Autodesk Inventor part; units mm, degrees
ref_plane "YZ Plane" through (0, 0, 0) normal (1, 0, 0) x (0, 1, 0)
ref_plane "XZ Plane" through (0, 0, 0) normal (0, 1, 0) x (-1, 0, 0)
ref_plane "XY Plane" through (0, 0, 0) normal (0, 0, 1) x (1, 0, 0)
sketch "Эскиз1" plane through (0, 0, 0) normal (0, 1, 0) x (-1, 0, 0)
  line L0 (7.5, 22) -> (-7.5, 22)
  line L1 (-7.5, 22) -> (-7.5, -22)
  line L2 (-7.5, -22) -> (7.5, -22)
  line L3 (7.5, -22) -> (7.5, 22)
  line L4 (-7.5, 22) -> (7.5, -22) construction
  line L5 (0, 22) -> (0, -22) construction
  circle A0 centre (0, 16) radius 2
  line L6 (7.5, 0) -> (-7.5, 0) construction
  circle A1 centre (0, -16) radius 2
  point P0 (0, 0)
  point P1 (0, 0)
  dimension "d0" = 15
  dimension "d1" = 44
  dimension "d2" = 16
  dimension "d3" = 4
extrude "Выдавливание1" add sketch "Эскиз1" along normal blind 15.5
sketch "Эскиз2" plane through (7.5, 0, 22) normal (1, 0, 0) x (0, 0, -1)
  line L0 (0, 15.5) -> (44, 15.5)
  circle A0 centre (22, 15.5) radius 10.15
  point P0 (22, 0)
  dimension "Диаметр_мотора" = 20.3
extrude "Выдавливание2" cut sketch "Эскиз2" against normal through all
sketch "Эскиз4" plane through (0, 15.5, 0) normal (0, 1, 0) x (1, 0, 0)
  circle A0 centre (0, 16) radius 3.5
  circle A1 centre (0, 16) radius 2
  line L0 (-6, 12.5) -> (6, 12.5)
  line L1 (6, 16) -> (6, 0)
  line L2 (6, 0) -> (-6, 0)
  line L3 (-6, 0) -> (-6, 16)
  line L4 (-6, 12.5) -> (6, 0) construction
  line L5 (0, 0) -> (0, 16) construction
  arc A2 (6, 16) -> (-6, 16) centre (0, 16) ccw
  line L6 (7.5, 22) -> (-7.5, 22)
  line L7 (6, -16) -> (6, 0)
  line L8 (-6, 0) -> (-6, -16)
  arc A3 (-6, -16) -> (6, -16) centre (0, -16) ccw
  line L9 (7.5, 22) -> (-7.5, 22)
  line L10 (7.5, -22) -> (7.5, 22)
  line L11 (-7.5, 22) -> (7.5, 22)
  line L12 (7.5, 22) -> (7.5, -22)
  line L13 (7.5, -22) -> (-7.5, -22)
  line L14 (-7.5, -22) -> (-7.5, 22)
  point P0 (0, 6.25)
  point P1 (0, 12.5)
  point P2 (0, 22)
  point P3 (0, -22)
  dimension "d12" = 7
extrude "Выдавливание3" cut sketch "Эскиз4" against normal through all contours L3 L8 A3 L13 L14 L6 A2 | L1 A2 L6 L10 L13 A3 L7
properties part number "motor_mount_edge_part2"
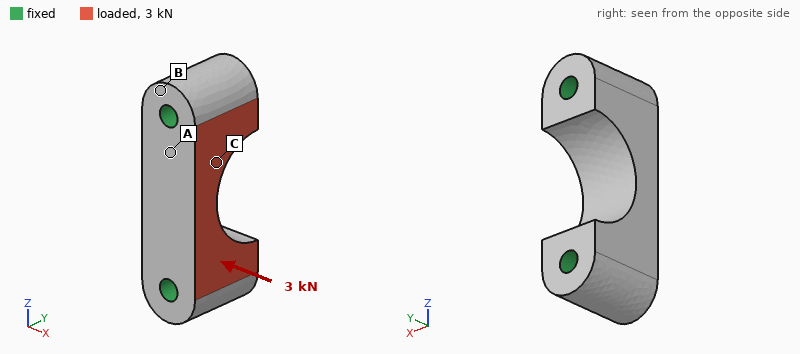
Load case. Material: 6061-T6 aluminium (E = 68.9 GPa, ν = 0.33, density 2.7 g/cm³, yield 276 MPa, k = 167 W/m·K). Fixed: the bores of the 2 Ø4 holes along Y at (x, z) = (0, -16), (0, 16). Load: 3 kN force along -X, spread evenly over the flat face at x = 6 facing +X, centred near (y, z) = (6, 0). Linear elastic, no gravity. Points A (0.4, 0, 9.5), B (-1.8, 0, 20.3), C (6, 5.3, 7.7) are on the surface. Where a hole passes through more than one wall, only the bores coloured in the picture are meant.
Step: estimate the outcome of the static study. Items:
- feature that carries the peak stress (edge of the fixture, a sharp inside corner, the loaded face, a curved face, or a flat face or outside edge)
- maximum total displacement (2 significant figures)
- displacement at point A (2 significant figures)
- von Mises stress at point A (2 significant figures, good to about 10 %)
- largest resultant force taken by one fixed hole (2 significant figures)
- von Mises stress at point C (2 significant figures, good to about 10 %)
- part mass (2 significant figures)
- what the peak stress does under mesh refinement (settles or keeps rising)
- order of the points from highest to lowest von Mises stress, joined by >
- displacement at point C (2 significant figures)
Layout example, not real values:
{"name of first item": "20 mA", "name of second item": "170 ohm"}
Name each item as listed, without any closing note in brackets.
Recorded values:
{"feature that carries the peak stress": "edge of the fixture", "maximum total displacement": "8.2 µm", "displacement at point A": "3.9 µm", "von Mises stress at point A": "19 MPa", "largest resultant force taken by one fixed hole": "1.5 kN", "von Mises stress at point C": "9.9 MPa", "part mass": "15 g", "what the peak stress does under mesh refinement": "keeps rising", "order of the points from highest to lowest von Mises stress, joined by >": "A > C > B", "displacement at point C": "5.2 µm"}
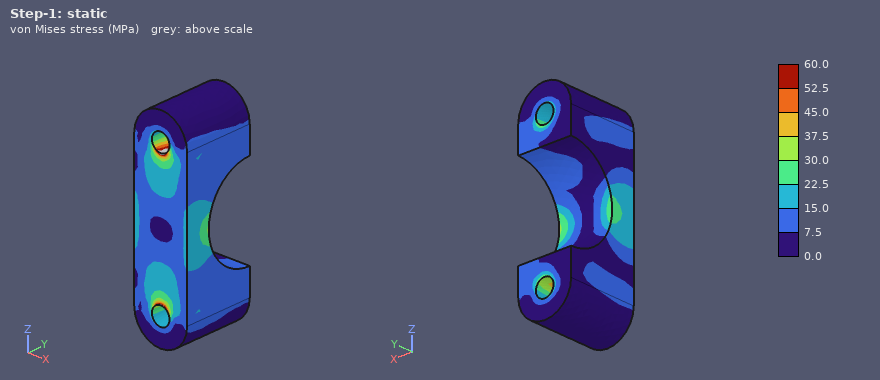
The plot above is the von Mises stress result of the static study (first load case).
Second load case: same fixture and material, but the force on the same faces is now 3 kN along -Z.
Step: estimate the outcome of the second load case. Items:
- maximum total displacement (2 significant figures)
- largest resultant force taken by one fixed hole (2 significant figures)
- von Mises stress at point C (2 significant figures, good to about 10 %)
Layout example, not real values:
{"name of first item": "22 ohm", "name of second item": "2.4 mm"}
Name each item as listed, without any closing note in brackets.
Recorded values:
{"maximum total displacement": "3.4 µm", "largest resultant force taken by one fixed hole": "1.5 kN", "von Mises stress at point C": "17 MPa"}
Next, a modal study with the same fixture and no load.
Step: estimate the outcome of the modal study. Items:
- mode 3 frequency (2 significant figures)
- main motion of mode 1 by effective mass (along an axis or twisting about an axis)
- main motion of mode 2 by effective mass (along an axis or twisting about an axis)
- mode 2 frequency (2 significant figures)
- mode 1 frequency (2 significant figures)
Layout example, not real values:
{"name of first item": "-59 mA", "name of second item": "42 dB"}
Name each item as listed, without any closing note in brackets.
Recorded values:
{"mode 3 frequency": "66 kHz", "main motion of mode 1 by effective mass": "along X", "main motion of mode 2 by effective mass": "along Y", "mode 2 frequency": "48 kHz", "mode 1 frequency": "36 kHz"}
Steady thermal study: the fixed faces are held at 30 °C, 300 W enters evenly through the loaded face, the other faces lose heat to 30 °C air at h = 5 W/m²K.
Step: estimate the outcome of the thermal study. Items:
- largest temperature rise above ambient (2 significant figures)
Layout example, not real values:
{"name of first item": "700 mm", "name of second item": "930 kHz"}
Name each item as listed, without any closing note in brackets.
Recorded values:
{"largest temperature rise above ambient": "64 K"}
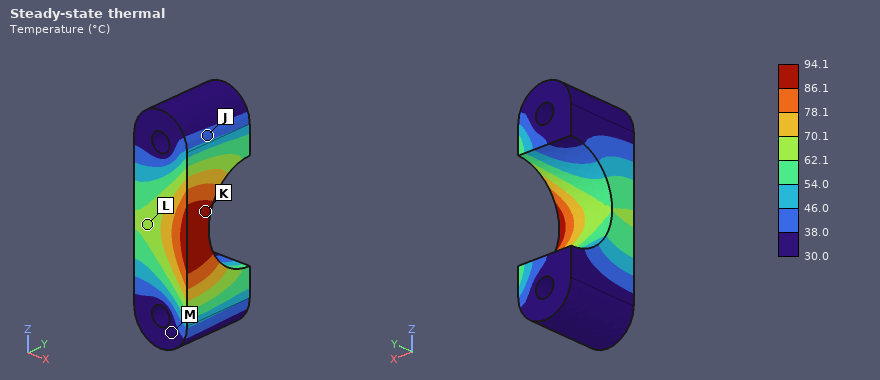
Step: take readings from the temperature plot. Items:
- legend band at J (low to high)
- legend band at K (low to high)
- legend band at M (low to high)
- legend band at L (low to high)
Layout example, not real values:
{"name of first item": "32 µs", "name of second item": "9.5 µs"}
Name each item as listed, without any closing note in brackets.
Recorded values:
{"legend band at J": "38.0 to 46.0 °C", "legend band at K": "86.1 to 94.1 °C", "legend band at M": "30.0 to 38.0 °C", "legend band at L": "62.1 to 70.1 °C"}
